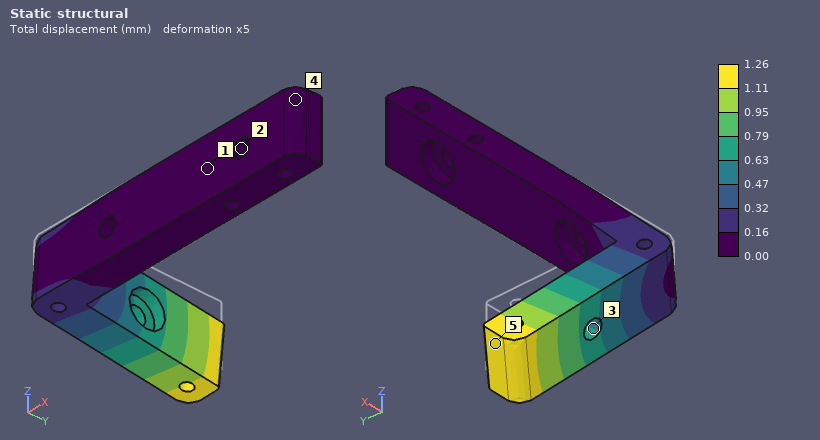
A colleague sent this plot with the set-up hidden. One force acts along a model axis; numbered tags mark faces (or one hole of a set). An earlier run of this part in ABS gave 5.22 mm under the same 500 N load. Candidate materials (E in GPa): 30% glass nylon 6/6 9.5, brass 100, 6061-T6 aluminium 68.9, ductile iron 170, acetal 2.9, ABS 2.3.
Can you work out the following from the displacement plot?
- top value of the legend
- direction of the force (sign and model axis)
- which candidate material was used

1.26 mm
-Z
30% glass nylon 6/6
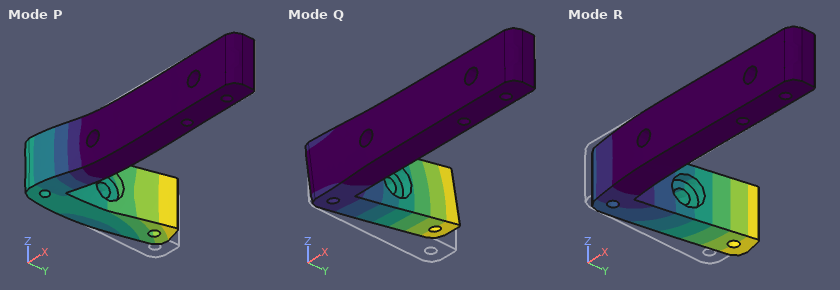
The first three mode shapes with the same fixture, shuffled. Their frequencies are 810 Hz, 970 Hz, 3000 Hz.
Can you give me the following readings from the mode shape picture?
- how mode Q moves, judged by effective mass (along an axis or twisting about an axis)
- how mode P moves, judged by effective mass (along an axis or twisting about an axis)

along Z
along Y
